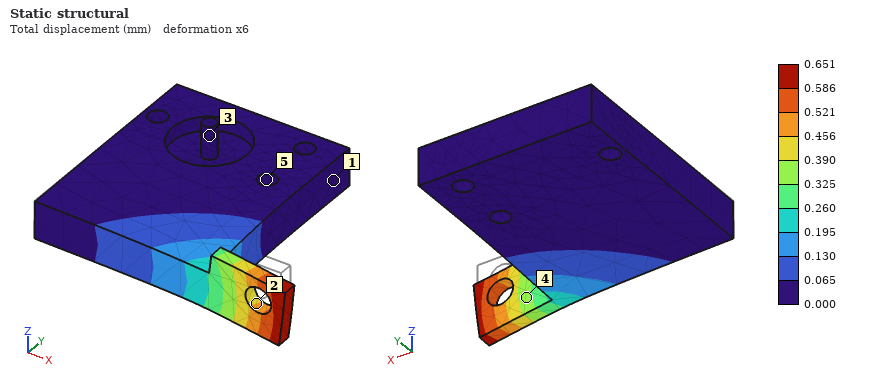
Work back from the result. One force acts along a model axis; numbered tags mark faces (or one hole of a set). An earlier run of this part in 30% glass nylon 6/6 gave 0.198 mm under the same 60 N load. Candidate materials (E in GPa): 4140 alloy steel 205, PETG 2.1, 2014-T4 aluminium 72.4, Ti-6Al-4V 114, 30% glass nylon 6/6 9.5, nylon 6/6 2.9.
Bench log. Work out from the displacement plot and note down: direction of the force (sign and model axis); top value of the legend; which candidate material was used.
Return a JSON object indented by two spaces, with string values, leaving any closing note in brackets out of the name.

{
  "direction of the force": "-Z",
  "top value of the legend": "0.651 mm",
  "which candidate material was used": "nylon 6/6"
}
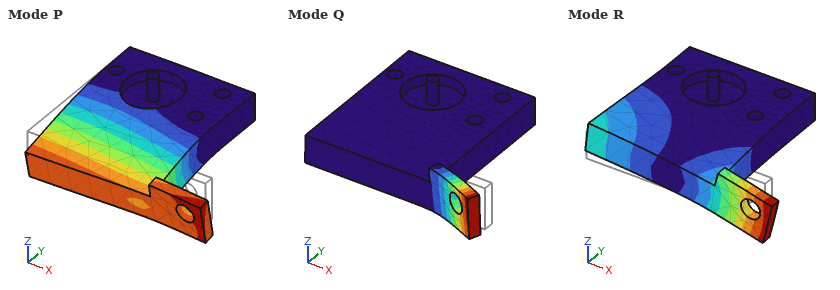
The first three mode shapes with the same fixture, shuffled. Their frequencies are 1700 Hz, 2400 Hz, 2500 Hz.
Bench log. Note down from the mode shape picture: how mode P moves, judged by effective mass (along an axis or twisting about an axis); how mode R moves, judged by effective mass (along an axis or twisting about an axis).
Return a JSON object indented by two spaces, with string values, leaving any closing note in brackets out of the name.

{
  "how mode P moves, judged by effective mass": "along Z",
  "how mode R moves, judged by effective mass": "twisting about Y"
}
